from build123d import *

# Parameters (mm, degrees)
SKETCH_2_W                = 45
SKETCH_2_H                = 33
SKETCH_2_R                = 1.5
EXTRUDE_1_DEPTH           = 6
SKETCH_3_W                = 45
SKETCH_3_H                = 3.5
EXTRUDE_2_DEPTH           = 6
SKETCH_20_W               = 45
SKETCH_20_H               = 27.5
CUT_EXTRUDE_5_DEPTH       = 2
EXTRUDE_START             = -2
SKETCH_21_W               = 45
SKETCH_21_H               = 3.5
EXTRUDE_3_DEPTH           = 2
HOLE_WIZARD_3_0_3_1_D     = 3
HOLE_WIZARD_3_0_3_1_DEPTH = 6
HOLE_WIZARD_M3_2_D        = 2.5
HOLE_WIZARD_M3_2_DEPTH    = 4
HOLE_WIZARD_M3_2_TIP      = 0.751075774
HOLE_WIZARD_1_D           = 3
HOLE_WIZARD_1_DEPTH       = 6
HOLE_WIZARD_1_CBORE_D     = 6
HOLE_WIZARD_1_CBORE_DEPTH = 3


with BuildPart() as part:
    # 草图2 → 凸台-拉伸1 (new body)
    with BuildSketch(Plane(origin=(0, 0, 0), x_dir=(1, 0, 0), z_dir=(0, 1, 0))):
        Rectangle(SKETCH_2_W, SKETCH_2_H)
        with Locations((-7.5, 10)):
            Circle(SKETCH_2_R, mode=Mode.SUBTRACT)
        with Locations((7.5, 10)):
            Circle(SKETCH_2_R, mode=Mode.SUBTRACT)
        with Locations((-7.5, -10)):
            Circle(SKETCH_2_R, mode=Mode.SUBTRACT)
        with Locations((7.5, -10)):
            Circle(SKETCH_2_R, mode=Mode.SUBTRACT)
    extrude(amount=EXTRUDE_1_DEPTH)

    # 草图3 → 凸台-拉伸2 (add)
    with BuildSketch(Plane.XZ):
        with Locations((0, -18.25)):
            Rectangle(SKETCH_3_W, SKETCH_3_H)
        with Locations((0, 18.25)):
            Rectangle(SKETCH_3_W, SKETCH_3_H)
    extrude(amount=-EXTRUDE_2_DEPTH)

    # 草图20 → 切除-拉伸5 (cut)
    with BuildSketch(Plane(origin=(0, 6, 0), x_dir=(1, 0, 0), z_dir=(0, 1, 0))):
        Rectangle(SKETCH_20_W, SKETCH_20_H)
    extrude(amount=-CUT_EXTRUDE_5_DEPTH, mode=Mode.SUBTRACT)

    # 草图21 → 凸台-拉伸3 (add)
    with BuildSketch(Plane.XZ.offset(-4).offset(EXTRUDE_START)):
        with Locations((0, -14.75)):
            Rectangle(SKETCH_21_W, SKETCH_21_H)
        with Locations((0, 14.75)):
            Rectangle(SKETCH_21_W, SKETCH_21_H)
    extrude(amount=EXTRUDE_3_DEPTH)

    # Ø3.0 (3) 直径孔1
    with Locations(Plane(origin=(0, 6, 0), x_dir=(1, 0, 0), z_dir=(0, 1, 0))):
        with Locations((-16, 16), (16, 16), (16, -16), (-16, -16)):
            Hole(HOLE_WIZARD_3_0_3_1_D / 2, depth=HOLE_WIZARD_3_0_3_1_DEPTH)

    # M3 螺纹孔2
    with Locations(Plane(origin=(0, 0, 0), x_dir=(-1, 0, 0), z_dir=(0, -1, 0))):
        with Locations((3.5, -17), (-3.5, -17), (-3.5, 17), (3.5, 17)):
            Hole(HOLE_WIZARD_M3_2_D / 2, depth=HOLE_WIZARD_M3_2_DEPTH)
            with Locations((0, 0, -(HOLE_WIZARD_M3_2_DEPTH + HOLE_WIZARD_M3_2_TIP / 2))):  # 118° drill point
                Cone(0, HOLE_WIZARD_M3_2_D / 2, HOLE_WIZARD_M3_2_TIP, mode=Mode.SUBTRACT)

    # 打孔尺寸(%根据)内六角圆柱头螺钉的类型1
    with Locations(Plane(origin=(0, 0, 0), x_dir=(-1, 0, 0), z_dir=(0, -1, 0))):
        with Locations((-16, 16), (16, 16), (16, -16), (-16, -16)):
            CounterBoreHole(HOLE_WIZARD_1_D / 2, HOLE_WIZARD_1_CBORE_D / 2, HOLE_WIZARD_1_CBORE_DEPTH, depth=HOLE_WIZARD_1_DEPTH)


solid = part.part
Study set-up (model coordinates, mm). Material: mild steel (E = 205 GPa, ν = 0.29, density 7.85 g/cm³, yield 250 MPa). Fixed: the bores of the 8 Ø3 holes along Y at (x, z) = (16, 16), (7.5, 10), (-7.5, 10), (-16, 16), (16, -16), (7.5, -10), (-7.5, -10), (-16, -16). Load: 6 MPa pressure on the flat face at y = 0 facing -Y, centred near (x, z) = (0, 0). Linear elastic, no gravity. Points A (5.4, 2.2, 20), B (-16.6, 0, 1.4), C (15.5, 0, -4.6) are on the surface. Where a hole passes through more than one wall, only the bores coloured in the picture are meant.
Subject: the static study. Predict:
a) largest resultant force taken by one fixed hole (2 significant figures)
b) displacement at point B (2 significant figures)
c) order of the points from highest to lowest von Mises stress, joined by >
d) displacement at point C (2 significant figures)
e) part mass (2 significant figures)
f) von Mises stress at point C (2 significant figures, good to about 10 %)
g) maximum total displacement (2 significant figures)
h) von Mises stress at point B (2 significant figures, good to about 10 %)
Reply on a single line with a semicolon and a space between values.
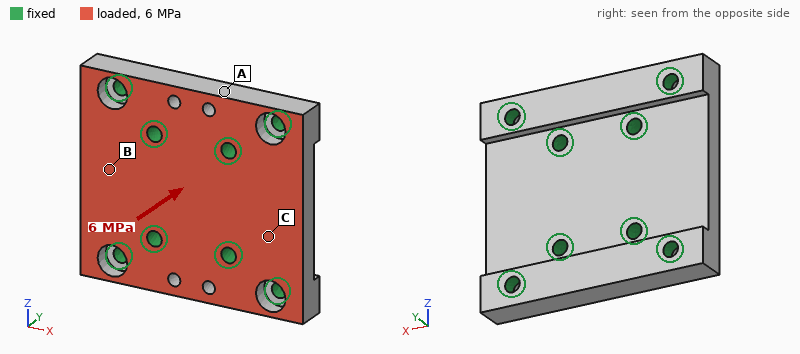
1.5 kN; 9.9 µm; B > C > A; 7.8 µm; 62 g; 42 MPa; 16 µm; 57 MPa
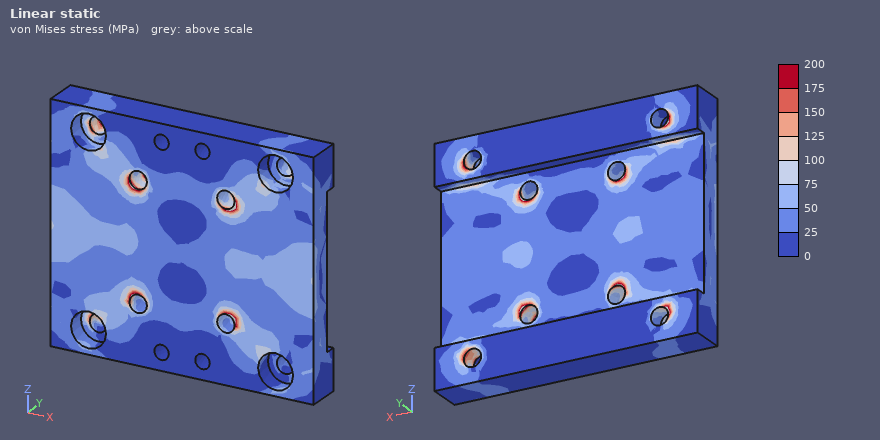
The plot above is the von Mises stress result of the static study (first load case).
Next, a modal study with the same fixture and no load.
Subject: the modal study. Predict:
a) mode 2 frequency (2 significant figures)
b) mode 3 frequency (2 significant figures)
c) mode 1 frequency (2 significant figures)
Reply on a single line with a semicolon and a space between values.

23 kHz; 34 kHz; 23 kHz
